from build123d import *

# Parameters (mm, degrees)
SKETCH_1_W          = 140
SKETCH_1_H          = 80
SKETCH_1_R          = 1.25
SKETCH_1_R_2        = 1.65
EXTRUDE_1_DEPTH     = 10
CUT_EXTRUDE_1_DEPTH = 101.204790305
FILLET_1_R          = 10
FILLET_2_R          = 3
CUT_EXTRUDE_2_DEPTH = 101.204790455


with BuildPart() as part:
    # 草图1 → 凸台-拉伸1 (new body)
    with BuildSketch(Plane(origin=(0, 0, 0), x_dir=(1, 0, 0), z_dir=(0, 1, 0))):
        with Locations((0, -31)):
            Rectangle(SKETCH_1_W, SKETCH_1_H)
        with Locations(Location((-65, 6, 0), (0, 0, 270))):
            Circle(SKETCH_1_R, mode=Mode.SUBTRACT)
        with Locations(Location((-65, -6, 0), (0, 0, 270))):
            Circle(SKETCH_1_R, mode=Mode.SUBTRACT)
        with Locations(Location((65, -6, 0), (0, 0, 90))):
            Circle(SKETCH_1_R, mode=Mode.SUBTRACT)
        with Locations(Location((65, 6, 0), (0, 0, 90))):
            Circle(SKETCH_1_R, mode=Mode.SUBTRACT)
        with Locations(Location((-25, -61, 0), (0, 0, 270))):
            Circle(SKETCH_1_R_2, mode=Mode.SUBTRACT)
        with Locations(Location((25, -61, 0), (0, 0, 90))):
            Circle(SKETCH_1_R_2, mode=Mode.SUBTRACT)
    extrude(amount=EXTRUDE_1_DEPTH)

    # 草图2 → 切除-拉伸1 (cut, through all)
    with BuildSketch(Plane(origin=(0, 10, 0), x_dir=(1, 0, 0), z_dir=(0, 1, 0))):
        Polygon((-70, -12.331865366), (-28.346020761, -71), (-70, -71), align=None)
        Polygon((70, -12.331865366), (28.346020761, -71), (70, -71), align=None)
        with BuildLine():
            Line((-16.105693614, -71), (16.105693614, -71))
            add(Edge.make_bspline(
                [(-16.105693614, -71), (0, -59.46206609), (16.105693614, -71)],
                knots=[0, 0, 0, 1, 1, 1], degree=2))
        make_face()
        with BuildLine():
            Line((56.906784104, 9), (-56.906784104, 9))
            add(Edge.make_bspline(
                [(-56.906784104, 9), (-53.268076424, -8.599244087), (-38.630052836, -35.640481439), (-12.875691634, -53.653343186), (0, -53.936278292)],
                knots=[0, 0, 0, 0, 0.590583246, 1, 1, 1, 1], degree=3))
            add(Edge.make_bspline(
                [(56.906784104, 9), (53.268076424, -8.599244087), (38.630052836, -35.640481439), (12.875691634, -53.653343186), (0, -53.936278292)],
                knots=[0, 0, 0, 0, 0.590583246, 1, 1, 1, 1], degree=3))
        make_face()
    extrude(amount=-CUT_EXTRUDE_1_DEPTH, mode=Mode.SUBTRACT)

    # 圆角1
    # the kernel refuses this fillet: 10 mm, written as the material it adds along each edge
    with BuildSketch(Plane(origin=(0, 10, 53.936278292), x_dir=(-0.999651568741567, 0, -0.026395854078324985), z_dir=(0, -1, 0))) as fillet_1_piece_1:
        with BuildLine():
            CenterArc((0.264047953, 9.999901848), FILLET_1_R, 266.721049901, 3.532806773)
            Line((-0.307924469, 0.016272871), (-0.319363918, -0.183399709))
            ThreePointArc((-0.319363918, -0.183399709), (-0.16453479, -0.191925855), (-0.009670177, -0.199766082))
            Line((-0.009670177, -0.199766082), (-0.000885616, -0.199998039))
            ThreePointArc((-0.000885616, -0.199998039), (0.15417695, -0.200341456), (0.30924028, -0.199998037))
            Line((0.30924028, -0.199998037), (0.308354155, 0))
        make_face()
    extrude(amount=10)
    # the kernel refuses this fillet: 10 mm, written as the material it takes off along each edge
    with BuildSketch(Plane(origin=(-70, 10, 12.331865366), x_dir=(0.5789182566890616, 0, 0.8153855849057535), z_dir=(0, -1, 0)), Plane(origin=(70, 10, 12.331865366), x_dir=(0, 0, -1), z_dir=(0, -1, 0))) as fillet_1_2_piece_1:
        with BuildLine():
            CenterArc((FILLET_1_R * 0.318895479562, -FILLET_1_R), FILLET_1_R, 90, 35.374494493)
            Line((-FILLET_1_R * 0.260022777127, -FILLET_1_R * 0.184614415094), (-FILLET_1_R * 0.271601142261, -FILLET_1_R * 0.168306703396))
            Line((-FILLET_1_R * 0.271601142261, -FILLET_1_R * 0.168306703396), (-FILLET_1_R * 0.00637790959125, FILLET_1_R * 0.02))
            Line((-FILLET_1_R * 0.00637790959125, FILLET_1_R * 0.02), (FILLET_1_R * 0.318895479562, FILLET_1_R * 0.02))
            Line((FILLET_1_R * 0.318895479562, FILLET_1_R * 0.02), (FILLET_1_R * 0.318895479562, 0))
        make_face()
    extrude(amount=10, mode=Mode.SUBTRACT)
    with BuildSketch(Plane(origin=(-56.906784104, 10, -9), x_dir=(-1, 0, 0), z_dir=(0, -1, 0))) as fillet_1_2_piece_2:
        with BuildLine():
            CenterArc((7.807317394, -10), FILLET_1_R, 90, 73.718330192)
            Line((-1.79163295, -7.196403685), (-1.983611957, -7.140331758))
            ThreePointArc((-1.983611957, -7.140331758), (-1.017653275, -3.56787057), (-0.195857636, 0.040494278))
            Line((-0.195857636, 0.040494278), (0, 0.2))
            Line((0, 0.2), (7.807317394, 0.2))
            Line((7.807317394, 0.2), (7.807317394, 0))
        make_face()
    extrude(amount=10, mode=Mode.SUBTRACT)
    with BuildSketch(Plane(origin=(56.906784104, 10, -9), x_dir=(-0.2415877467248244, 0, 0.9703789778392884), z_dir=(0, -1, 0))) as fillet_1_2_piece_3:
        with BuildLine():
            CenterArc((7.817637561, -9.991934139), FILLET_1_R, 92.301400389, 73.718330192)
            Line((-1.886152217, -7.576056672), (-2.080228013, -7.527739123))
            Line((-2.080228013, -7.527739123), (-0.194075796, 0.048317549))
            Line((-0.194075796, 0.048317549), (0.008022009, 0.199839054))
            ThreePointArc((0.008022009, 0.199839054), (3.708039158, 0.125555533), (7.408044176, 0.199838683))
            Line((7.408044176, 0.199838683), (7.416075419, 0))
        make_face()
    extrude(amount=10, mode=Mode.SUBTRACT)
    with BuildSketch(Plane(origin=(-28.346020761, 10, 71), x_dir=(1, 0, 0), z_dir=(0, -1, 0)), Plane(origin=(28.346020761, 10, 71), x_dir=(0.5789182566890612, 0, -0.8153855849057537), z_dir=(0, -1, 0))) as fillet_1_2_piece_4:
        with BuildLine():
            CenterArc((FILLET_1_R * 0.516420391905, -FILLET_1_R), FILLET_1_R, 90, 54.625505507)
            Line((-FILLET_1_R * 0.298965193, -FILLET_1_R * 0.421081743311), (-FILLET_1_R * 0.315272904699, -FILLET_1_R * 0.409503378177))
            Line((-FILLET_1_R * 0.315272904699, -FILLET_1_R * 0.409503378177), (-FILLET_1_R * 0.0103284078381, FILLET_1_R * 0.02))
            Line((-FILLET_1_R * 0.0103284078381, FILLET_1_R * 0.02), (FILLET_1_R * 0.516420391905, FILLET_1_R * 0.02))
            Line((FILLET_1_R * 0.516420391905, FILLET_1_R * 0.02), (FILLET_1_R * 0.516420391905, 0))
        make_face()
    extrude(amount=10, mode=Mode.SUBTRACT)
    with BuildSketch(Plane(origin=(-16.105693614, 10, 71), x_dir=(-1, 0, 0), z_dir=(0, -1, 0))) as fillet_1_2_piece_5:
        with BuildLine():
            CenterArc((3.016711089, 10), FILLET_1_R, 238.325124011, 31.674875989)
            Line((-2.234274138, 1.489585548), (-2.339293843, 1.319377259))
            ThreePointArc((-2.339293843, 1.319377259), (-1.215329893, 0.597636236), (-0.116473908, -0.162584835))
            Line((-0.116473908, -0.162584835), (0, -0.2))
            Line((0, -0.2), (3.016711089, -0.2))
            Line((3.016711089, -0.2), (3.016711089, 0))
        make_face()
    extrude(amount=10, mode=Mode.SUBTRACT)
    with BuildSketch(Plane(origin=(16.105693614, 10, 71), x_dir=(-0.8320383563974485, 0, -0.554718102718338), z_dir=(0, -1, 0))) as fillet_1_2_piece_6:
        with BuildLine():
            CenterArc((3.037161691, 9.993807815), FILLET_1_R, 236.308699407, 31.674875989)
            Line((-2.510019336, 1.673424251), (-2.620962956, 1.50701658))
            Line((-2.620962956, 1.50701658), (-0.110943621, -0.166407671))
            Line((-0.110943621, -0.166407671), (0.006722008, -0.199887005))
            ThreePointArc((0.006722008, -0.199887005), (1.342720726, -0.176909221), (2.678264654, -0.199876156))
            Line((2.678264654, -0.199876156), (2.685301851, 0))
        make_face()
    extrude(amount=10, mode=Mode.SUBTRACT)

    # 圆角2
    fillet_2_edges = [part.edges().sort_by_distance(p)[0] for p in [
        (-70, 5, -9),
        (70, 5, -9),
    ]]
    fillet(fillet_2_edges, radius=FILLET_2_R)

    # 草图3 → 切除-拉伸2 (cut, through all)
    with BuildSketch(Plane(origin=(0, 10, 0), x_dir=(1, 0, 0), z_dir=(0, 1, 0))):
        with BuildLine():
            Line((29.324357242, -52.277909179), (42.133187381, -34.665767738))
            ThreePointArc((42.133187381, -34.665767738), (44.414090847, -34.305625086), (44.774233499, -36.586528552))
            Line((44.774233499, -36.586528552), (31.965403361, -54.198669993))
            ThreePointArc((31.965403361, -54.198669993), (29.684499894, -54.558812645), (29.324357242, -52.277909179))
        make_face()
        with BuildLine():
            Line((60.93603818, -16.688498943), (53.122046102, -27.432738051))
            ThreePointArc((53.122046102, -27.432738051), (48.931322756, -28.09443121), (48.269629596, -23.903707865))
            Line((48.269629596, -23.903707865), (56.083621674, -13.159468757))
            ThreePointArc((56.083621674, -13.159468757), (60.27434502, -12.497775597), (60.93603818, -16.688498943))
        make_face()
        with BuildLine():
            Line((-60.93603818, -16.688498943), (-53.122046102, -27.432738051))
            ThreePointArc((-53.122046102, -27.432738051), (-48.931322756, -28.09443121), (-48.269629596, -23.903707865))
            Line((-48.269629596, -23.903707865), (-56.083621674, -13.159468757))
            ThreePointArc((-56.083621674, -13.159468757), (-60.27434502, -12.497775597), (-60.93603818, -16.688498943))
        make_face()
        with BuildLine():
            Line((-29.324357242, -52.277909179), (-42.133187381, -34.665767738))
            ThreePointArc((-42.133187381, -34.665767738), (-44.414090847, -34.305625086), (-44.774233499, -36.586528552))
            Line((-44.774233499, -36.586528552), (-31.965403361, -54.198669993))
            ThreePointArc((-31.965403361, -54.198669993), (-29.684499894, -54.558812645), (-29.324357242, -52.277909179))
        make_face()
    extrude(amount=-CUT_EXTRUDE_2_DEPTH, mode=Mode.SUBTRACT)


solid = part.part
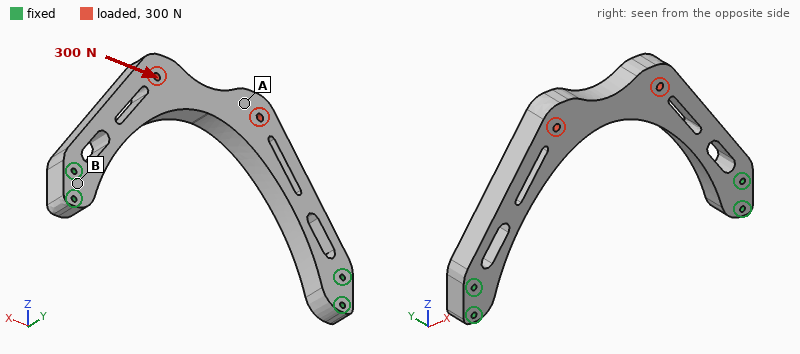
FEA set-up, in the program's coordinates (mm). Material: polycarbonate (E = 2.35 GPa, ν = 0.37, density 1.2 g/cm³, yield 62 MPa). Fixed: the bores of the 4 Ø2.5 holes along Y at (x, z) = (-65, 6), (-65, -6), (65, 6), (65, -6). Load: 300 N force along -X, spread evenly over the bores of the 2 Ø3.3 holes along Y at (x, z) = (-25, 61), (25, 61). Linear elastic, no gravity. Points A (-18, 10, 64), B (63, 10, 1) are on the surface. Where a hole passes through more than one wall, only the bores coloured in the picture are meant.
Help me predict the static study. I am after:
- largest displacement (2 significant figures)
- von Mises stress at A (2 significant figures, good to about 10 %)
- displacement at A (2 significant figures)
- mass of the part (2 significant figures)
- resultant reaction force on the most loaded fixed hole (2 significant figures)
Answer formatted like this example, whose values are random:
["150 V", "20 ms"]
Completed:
["0.26 mm", "1.7 MPa", "0.22 mm", "37 g", "260 N"]
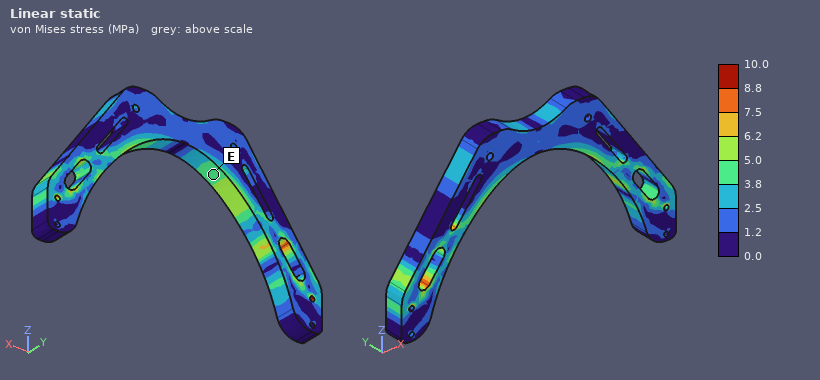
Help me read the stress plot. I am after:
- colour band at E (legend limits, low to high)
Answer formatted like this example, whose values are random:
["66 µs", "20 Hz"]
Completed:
["3.8 to 5.0 MPa"]
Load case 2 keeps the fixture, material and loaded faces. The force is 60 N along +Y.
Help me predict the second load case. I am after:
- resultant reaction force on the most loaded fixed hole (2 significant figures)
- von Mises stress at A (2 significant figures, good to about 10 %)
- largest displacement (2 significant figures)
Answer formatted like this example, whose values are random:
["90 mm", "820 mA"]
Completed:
["76 N", "1.1 MPa", "1.5 mm"]
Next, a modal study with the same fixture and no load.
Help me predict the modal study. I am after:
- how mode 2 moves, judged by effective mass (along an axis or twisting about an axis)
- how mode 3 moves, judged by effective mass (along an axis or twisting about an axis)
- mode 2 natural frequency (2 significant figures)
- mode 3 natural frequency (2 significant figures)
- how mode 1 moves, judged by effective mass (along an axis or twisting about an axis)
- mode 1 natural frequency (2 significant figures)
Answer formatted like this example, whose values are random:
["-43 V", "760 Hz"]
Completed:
["twisting about Z", "along X", "830 Hz", "1100 Hz", "along Y", "270 Hz"]
